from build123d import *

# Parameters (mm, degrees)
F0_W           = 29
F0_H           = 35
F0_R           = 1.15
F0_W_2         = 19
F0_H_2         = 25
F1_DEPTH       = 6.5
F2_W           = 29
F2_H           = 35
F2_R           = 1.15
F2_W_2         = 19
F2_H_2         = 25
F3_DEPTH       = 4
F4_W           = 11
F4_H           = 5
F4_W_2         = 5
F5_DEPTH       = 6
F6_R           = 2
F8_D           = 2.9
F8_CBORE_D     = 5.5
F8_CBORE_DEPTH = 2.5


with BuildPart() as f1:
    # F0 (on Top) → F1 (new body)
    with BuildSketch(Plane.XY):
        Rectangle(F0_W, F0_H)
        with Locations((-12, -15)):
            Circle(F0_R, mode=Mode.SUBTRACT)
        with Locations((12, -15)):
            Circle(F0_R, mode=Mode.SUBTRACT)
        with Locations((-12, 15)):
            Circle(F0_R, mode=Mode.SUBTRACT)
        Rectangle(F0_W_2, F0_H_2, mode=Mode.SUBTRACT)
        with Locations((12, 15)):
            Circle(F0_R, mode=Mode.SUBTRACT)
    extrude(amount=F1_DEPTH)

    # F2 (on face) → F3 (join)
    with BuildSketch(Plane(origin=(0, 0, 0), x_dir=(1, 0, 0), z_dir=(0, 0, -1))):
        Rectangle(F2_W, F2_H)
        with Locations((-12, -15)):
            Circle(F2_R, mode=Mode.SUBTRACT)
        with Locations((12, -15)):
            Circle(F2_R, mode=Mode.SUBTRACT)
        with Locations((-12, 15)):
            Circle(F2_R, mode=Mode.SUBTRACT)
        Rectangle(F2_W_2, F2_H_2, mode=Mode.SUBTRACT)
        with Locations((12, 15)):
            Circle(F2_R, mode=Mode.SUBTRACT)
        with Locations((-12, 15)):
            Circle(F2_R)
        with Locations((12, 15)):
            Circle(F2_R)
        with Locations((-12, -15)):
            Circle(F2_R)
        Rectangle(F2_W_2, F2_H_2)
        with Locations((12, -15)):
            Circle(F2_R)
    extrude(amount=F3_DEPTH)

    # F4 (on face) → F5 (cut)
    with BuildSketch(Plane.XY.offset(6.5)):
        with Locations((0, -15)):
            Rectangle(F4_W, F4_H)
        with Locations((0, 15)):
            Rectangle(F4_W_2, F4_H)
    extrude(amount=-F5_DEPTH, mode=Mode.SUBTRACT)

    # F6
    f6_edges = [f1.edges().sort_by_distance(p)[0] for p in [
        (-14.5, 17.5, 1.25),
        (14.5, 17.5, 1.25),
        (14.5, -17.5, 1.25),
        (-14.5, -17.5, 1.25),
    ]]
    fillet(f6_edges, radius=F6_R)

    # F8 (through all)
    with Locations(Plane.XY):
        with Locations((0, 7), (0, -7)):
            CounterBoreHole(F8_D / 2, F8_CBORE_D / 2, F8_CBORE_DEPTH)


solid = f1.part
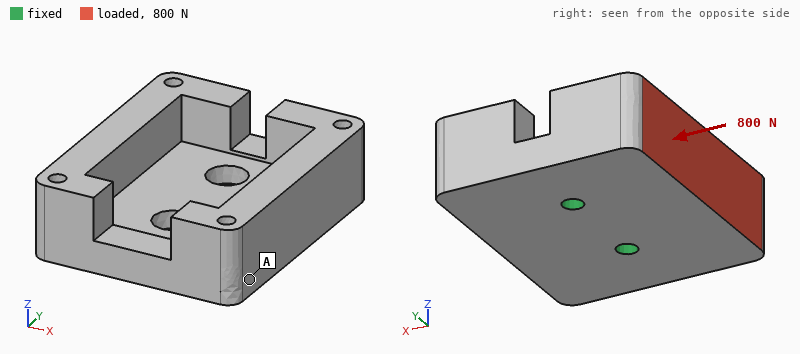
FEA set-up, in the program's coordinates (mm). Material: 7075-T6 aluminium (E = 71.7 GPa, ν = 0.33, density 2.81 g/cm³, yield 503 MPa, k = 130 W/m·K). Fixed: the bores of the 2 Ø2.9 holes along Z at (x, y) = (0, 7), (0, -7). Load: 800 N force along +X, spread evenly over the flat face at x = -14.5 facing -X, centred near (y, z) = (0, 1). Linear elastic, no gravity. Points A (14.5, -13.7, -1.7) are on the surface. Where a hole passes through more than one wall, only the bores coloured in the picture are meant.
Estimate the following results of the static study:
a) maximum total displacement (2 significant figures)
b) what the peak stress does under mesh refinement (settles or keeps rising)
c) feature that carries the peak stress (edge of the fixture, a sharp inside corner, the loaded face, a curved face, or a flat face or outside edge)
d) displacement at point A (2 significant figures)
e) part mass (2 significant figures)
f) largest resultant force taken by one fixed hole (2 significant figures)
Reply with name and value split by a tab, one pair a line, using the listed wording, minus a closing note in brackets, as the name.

maximum total displacement	87 µm
what the peak stress does under mesh refinement	keeps rising
feature that carries the peak stress	edge of the fixture
displacement at point A	54 µm
part mass	19 g
largest resultant force taken by one fixed hole	400 N
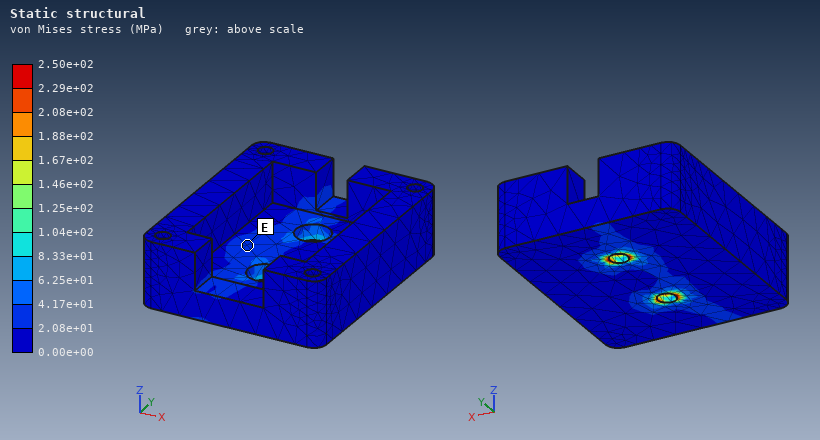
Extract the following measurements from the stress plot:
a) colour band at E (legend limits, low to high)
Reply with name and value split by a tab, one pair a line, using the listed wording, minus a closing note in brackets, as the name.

colour band at E	2.08e+01 to 4.17e+01 MPa
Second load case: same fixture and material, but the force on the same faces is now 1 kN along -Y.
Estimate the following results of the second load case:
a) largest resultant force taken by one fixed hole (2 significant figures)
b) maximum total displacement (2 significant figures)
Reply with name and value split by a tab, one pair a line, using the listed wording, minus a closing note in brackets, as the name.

largest resultant force taken by one fixed hole	1.1 kN
maximum total displacement	25 µm
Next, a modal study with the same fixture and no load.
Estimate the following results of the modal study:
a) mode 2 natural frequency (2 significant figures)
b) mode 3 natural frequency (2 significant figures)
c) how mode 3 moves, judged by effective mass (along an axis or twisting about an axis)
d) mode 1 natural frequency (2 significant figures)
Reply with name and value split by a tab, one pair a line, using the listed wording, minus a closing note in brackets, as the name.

mode 2 natural frequency	8400 Hz
mode 3 natural frequency	9100 Hz
how mode 3 moves, judged by effective mass	along Z
mode 1 natural frequency	3200 Hz
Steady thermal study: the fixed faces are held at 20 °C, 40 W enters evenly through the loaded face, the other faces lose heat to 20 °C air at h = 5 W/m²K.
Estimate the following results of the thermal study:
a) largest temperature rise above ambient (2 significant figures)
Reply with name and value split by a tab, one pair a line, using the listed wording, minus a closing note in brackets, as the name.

largest temperature rise above ambient	43 K
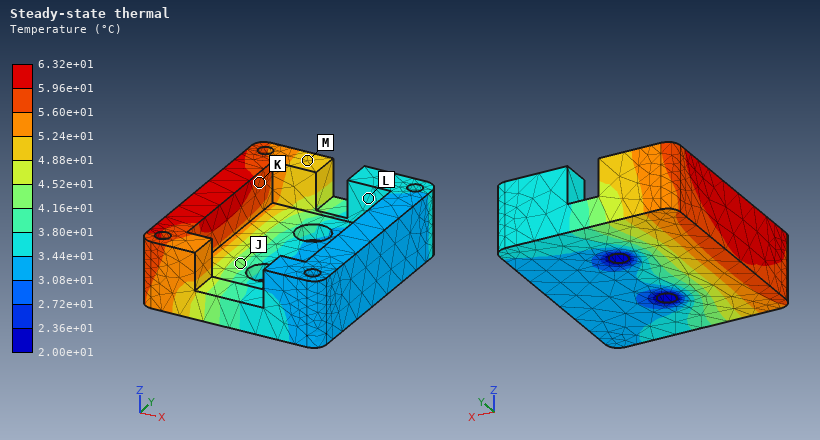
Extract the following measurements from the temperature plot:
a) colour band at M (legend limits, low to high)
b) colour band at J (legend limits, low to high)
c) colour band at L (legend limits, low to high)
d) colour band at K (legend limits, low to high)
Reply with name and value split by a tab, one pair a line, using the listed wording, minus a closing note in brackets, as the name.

colour band at M	4.88e+01 to 5.24e+01 °C
colour band at J	4.16e+01 to 4.52e+01 °C
colour band at L	3.44e+01 to 3.80e+01 °C
colour band at K	5.60e+01 to 5.96e+01 °C
